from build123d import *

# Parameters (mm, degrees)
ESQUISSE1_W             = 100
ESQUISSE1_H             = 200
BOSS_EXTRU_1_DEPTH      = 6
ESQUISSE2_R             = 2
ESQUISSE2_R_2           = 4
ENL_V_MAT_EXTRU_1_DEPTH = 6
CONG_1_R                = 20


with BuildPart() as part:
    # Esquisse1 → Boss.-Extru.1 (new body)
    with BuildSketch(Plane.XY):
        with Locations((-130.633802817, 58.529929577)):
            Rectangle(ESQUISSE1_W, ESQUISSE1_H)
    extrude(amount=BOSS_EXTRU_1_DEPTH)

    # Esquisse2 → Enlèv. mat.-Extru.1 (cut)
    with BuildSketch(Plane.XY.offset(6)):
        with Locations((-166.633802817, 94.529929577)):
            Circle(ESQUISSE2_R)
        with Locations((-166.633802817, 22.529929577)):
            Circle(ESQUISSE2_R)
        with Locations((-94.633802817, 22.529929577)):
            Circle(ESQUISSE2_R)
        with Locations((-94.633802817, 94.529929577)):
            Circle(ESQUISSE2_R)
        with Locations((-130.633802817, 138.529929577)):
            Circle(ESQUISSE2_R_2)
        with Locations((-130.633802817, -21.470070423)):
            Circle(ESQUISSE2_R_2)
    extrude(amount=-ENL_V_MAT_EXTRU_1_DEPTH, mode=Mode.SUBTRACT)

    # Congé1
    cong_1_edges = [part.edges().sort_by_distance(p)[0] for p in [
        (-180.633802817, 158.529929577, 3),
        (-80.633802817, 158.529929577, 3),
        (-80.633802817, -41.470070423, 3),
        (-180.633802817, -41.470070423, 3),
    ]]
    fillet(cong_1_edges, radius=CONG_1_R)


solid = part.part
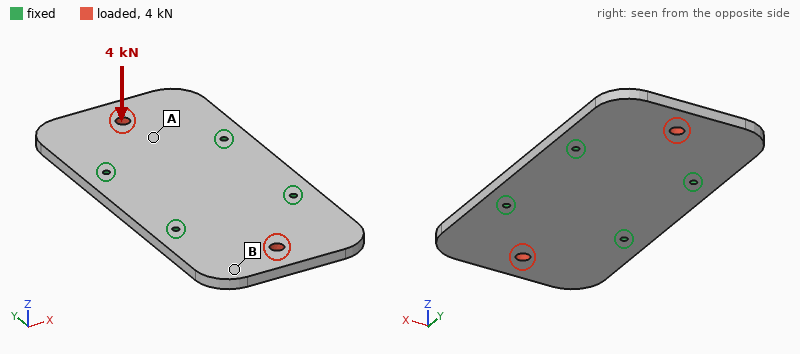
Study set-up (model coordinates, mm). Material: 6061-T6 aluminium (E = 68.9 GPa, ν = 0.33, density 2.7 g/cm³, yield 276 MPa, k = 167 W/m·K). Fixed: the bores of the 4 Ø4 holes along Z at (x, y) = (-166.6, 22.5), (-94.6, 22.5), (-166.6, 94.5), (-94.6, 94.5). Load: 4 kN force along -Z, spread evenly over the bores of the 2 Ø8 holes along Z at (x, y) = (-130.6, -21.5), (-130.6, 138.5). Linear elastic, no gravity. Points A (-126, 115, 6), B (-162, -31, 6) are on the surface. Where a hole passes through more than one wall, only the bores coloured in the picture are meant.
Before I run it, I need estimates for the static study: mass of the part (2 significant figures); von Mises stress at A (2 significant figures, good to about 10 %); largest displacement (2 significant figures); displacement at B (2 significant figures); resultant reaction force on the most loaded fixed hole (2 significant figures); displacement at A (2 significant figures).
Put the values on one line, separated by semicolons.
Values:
320 g; 86 MPa; 1.2 mm; 0.85 mm; 1.0 kN; 0.32 mm
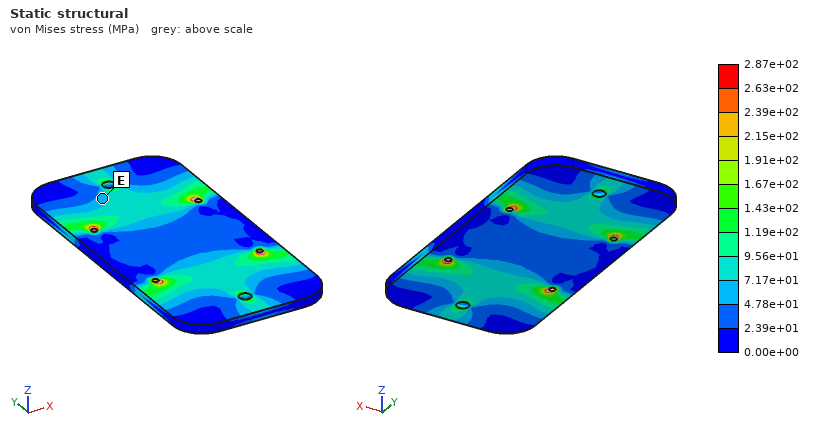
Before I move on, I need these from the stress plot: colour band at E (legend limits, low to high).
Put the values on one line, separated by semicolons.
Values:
4.78e+01 to 7.17e+01 MPa
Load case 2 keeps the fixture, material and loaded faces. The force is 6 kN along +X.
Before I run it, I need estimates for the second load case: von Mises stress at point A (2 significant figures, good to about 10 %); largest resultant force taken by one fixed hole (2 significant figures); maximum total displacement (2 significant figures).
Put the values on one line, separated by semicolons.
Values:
11 MPa; 2.0 kN; 19 µm
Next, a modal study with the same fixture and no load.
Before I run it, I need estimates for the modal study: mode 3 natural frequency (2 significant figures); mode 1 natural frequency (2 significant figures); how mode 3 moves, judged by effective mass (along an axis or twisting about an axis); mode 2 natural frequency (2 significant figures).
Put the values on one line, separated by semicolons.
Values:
2200 Hz; 1100 Hz; twisting about Y; 1100 Hz
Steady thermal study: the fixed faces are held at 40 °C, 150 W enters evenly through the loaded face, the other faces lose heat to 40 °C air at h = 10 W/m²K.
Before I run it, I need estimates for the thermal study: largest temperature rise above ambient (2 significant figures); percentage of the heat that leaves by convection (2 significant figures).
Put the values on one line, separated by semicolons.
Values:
63 K; 6.4 %
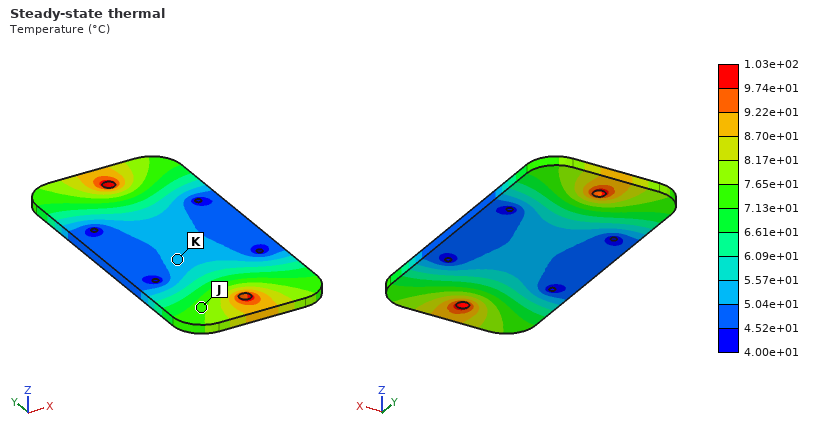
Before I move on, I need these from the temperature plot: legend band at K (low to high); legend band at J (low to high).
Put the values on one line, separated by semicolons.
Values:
5.04e+01 to 5.57e+01 °C; 7.13e+01 to 7.65e+01 °C
